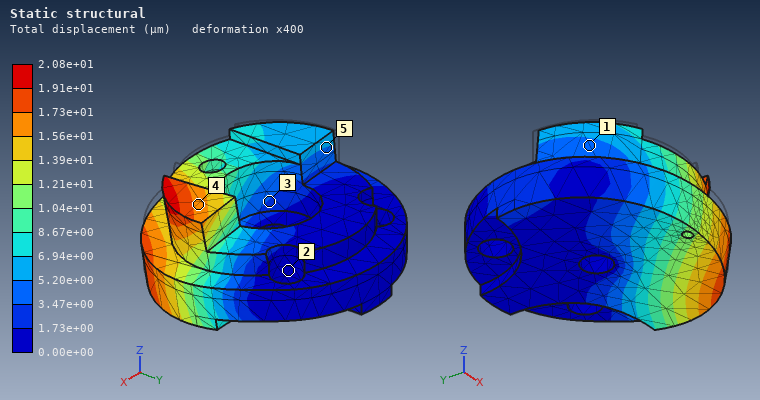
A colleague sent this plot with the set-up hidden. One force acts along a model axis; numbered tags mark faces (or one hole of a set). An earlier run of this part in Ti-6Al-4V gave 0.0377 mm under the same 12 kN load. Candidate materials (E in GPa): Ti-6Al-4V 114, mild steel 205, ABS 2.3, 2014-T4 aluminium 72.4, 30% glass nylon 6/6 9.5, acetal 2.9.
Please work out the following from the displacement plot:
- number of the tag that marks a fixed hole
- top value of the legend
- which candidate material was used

2
2.08e+01 µm
mild steel
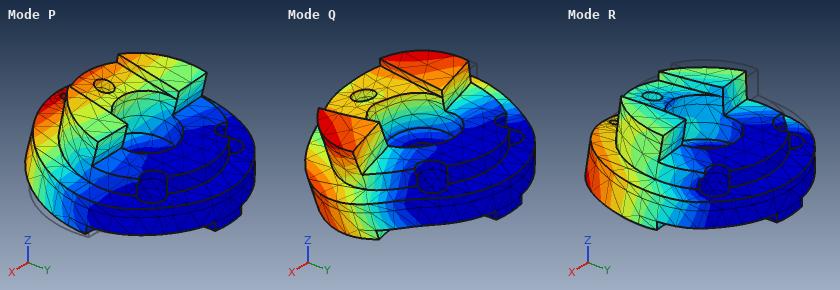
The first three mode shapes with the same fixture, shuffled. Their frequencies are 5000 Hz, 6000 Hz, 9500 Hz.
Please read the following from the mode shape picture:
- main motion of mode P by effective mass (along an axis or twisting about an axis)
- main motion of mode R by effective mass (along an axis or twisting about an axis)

along Z
along X
